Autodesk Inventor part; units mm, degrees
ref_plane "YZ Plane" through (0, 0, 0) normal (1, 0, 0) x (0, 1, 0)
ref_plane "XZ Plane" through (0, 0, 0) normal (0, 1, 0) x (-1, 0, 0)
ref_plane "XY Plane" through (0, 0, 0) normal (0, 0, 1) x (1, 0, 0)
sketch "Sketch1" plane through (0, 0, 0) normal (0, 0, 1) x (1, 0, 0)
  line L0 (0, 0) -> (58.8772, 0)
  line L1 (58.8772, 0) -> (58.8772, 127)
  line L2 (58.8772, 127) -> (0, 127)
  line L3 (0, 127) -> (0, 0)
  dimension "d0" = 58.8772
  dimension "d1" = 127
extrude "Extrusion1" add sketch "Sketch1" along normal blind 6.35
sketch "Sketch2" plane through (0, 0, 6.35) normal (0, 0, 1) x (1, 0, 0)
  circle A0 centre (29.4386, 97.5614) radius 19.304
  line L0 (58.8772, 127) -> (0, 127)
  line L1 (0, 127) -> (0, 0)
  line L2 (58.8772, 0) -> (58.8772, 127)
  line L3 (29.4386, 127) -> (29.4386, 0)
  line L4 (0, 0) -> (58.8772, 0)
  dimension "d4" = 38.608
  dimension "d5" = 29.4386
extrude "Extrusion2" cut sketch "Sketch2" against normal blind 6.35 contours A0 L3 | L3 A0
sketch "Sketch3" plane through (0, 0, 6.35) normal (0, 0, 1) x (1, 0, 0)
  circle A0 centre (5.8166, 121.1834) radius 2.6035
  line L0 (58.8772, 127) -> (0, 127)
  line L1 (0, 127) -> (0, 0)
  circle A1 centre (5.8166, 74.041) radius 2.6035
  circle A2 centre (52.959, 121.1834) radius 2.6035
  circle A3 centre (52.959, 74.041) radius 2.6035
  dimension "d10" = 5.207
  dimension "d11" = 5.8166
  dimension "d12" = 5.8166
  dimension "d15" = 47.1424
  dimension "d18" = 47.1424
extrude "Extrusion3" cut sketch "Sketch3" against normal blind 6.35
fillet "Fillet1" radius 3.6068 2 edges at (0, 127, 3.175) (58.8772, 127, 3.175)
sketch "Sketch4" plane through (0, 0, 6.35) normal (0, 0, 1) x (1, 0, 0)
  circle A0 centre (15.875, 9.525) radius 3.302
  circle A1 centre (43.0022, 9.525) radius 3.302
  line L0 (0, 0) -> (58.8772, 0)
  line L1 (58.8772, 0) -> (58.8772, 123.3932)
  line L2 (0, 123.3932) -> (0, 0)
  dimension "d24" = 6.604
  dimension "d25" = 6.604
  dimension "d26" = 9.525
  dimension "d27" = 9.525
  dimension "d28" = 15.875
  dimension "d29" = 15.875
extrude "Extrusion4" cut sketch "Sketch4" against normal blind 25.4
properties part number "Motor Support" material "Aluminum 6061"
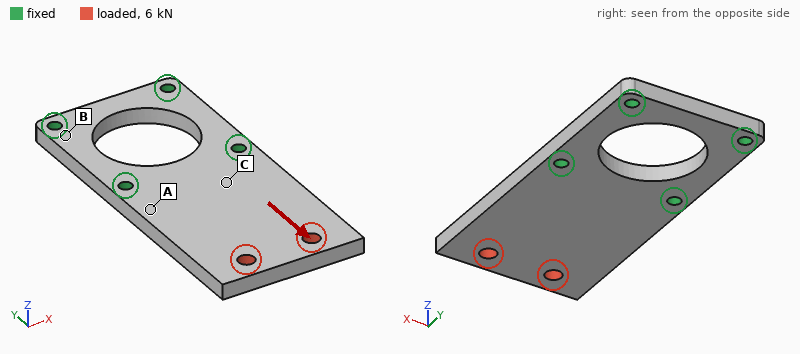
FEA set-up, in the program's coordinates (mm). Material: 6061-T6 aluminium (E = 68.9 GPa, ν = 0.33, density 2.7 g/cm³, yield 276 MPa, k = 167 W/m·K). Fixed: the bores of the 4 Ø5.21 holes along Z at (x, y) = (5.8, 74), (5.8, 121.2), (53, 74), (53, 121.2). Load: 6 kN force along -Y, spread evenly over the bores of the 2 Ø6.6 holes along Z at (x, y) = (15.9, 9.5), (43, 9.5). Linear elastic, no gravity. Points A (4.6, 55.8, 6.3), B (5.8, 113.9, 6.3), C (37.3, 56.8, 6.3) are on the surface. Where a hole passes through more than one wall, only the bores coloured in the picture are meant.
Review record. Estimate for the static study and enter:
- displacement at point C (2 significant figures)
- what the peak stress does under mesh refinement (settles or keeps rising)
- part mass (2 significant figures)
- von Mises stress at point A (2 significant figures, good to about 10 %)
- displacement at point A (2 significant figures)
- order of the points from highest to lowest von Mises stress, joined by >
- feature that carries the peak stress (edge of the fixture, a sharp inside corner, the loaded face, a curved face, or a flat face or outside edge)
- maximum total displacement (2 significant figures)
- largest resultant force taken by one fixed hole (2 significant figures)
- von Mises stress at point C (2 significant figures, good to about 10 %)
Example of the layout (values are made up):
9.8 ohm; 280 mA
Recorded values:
8.2 µm; keeps rising; 110 g; 22 MPa; 6.7 µm; A > C > B; edge of the fixture; 23 µm; 3.0 kN; 12 MPa
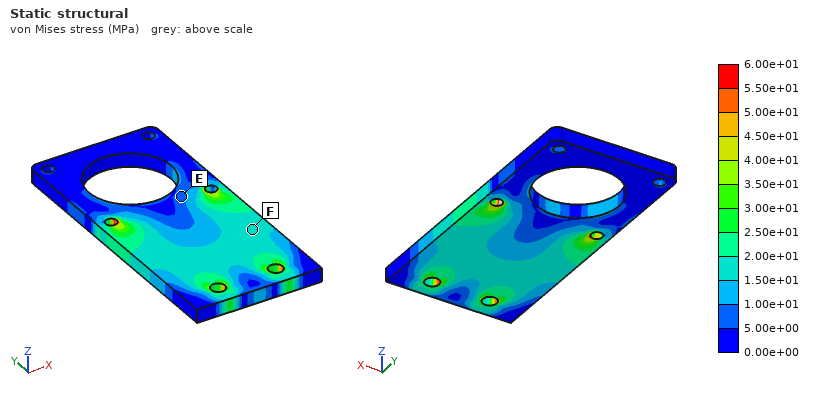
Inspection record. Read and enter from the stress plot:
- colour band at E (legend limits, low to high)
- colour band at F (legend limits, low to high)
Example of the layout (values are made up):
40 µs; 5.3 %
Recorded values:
5.00e+00 to 1.00e+01 MPa; 1.50e+01 to 2.00e+01 MPa
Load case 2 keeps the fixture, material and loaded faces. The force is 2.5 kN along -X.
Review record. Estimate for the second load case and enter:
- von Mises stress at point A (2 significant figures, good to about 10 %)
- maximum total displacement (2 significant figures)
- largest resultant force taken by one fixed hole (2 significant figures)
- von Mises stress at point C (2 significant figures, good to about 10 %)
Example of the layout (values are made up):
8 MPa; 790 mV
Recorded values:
28 MPa; 63 µm; 3.5 kN; 16 MPa
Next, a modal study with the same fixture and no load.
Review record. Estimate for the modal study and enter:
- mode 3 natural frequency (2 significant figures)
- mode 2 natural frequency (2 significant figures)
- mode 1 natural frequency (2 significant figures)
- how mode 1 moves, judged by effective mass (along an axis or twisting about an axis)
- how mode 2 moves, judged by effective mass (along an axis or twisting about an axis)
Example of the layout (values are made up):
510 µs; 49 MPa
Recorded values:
5500 Hz; 2700 Hz; 890 Hz; along Z; twisting about Y
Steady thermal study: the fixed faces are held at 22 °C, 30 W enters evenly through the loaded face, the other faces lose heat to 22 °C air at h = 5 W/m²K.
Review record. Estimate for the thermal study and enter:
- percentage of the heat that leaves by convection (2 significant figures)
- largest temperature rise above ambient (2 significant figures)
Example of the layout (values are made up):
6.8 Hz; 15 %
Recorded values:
3.3 %; 36 K
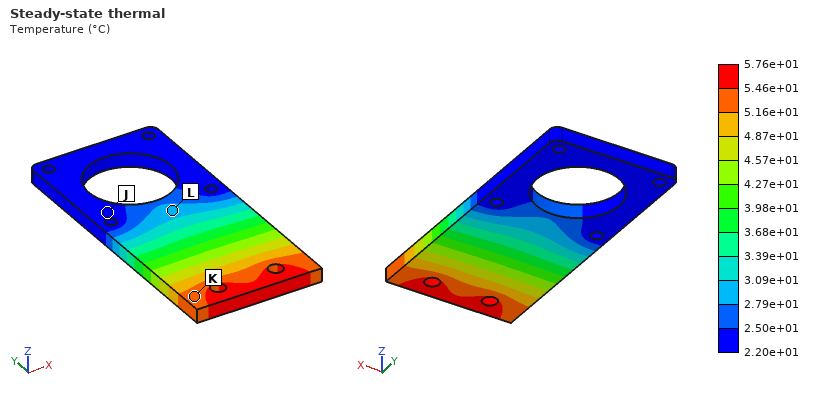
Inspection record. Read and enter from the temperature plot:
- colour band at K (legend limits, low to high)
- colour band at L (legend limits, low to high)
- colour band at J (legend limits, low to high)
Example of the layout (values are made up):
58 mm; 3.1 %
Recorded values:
5.16e+01 to 5.46e+01 °C; 2.79e+01 to 3.09e+01 °C; 2.20e+01 to 2.50e+01 °C
